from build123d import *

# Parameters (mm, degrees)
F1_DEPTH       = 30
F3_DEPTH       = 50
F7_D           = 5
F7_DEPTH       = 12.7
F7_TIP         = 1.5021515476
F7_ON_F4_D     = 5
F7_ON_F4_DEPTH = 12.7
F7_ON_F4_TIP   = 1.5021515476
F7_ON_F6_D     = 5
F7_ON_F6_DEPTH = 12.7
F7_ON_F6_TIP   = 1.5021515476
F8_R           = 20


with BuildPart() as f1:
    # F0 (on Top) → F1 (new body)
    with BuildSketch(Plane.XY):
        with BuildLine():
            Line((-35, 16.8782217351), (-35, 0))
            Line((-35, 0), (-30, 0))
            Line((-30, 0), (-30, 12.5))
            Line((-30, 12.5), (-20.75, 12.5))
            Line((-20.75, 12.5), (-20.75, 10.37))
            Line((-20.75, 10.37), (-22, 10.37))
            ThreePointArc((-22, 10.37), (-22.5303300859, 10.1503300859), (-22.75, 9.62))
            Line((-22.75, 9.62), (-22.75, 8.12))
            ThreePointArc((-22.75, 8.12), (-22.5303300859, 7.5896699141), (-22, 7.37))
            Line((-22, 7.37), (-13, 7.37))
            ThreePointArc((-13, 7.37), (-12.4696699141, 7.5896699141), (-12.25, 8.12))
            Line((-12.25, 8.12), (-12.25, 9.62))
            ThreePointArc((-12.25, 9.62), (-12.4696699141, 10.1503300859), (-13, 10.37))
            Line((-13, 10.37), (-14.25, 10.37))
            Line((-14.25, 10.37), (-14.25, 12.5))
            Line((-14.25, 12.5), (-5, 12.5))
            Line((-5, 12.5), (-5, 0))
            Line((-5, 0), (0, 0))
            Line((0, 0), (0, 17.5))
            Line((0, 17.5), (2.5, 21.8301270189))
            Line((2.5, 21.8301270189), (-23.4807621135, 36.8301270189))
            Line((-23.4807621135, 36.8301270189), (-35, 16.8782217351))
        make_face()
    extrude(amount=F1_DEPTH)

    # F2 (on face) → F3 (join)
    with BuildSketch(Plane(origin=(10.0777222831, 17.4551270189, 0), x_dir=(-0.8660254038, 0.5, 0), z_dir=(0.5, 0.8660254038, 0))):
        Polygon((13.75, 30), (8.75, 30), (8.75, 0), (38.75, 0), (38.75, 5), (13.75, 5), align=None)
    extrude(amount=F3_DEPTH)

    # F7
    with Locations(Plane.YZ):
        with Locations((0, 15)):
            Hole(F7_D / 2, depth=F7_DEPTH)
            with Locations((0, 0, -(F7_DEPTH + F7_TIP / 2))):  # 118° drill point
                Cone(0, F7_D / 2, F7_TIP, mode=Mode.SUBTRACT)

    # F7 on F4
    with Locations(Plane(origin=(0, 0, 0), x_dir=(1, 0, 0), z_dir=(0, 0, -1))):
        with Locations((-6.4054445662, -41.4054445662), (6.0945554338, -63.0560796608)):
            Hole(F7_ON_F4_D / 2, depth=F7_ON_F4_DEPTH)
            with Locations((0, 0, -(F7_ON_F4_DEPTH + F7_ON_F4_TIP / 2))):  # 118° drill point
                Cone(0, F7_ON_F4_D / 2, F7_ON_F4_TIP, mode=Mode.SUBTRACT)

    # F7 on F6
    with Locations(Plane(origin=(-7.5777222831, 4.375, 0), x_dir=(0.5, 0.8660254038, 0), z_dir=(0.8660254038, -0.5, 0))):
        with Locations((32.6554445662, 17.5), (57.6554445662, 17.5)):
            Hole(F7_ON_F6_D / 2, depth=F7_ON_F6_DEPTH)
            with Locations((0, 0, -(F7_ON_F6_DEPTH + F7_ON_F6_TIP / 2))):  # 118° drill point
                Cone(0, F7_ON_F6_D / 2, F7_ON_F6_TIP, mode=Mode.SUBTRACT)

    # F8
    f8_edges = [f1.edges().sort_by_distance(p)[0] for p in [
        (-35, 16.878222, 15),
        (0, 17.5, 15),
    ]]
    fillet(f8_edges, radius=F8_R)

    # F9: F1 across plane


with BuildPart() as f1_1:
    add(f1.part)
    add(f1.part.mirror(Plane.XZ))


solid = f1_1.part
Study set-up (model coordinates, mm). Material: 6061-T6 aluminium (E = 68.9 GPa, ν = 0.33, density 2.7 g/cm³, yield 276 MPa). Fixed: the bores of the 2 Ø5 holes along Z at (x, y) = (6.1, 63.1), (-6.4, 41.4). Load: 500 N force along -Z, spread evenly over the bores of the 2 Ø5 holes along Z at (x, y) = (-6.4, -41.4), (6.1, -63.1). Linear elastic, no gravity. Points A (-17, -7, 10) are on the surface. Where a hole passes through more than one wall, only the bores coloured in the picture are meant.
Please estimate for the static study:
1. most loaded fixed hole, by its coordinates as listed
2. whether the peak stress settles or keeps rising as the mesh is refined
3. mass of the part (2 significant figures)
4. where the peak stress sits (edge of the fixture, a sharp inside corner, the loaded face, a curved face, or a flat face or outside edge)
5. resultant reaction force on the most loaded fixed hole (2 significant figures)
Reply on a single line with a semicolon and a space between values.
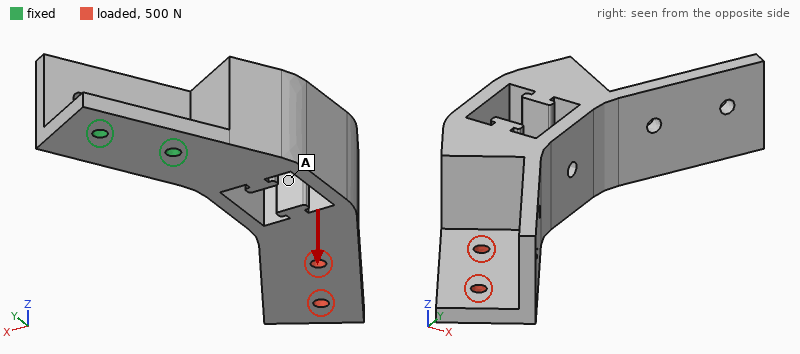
(-6.4, 41.4); keeps rising; 190 g; edge of the fixture; 1.6 kN
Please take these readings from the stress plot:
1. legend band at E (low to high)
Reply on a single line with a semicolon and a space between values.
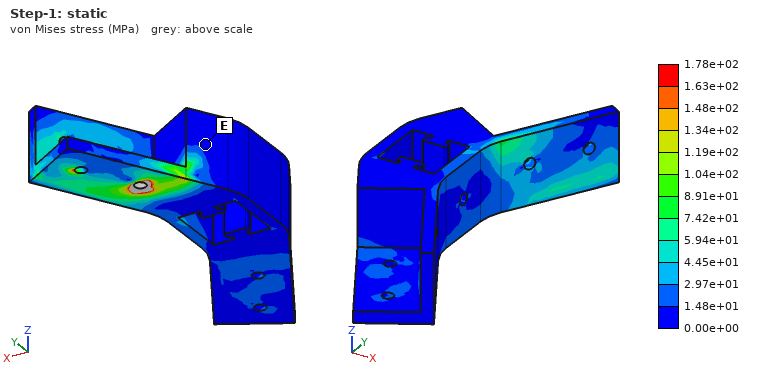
0.00e+00 to 1.48e+01 MPa
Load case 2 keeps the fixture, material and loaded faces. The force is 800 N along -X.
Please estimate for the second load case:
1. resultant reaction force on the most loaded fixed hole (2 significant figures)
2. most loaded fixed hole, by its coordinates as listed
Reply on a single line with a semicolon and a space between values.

3.1 kN; (-6.4, 41.4)
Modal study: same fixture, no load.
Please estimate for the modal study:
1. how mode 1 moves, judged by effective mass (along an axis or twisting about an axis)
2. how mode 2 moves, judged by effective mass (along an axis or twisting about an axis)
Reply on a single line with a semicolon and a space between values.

along Z; along X
